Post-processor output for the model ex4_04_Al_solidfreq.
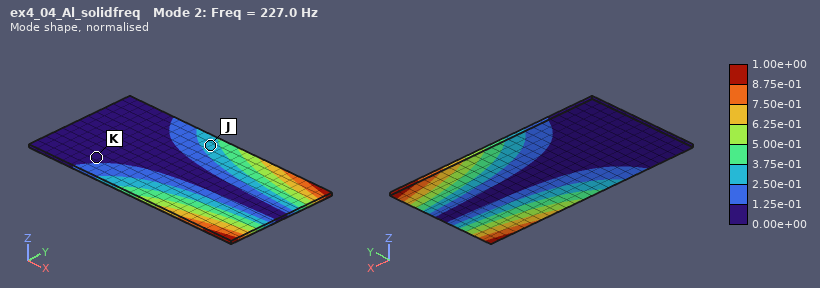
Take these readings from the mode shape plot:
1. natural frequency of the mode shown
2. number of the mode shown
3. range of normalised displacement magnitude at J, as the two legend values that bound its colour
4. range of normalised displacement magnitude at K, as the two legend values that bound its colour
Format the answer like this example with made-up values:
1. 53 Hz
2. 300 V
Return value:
1. 227.0 Hz
2. 2
3. 2.50e-01 to 3.75e-01
4. 0.00e+00 to 1.25e-01
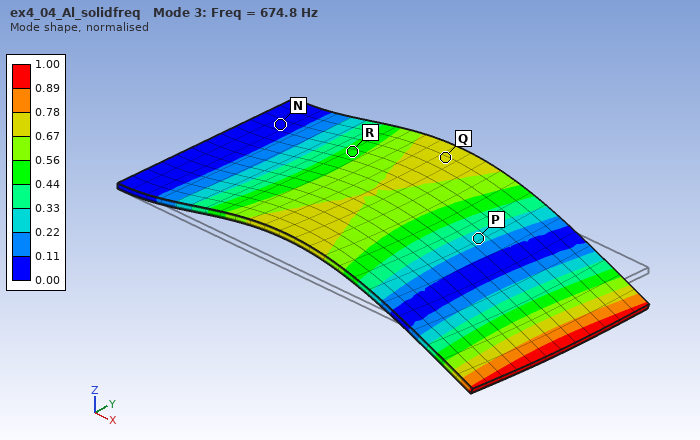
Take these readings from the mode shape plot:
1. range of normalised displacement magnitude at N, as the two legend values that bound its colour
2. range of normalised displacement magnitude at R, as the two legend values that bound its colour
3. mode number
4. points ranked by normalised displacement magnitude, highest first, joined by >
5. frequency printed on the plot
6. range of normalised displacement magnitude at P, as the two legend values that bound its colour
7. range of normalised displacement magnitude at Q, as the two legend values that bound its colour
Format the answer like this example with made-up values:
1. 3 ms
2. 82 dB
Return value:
1. 0.00 to 0.11
2. 0.44 to 0.56
3. 3
4. Q > R > P > N
5. 674.8 Hz
6. 0.22 to 0.33
7. 0.67 to 0.78
